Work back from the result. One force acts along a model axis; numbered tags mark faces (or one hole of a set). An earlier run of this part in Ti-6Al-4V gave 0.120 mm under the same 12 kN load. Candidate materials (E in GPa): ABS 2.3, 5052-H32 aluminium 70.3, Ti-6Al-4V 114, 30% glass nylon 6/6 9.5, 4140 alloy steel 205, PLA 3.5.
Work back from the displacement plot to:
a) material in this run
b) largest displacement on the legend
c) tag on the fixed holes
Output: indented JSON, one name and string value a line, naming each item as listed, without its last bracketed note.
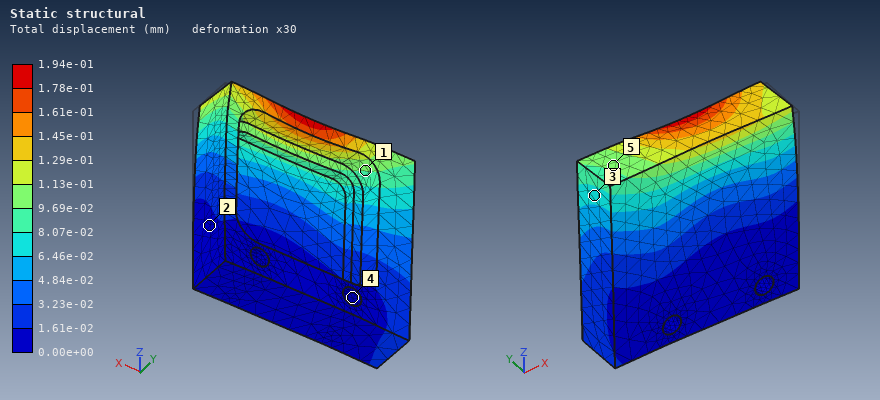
{
  "material in this run": "5052-H32 aluminium",
  "largest displacement on the legend": "1.94e-01 mm",
  "tag on the fixed holes": "4"
}
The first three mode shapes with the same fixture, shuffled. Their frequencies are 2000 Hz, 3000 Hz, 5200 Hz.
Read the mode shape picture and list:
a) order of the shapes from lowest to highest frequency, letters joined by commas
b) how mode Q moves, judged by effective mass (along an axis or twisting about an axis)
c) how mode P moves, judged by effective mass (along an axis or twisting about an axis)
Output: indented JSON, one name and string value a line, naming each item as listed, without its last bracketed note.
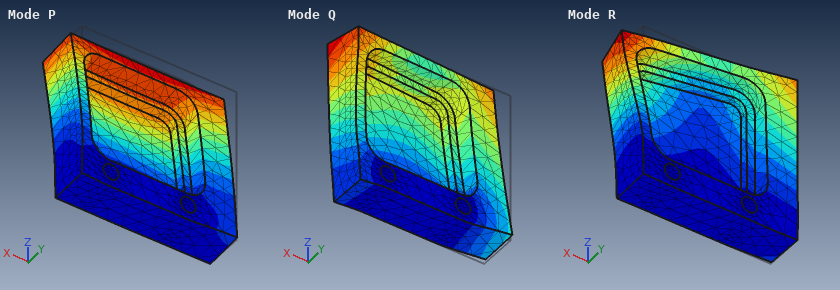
{
  "order of the shapes from lowest to highest frequency, letters joined by commas": "P, R, Q",
  "how mode Q moves, judged by effective mass": "along X",
  "how mode P moves, judged by effective mass": "along Y"
}
